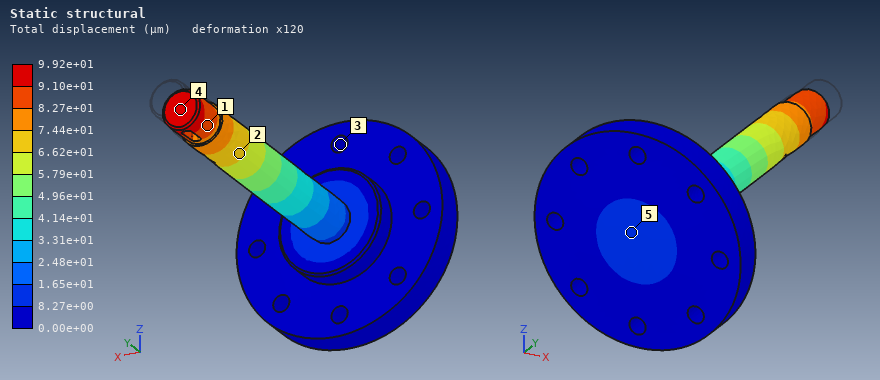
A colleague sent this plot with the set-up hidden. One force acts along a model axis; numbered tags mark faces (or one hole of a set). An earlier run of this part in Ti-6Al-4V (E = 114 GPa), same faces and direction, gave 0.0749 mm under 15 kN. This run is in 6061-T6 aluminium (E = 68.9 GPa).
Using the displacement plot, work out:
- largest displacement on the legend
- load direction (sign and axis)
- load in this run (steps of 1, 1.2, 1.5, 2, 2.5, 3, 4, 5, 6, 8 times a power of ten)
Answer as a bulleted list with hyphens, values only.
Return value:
- 9.92e+01 µm
- -Y
- 12 kN
